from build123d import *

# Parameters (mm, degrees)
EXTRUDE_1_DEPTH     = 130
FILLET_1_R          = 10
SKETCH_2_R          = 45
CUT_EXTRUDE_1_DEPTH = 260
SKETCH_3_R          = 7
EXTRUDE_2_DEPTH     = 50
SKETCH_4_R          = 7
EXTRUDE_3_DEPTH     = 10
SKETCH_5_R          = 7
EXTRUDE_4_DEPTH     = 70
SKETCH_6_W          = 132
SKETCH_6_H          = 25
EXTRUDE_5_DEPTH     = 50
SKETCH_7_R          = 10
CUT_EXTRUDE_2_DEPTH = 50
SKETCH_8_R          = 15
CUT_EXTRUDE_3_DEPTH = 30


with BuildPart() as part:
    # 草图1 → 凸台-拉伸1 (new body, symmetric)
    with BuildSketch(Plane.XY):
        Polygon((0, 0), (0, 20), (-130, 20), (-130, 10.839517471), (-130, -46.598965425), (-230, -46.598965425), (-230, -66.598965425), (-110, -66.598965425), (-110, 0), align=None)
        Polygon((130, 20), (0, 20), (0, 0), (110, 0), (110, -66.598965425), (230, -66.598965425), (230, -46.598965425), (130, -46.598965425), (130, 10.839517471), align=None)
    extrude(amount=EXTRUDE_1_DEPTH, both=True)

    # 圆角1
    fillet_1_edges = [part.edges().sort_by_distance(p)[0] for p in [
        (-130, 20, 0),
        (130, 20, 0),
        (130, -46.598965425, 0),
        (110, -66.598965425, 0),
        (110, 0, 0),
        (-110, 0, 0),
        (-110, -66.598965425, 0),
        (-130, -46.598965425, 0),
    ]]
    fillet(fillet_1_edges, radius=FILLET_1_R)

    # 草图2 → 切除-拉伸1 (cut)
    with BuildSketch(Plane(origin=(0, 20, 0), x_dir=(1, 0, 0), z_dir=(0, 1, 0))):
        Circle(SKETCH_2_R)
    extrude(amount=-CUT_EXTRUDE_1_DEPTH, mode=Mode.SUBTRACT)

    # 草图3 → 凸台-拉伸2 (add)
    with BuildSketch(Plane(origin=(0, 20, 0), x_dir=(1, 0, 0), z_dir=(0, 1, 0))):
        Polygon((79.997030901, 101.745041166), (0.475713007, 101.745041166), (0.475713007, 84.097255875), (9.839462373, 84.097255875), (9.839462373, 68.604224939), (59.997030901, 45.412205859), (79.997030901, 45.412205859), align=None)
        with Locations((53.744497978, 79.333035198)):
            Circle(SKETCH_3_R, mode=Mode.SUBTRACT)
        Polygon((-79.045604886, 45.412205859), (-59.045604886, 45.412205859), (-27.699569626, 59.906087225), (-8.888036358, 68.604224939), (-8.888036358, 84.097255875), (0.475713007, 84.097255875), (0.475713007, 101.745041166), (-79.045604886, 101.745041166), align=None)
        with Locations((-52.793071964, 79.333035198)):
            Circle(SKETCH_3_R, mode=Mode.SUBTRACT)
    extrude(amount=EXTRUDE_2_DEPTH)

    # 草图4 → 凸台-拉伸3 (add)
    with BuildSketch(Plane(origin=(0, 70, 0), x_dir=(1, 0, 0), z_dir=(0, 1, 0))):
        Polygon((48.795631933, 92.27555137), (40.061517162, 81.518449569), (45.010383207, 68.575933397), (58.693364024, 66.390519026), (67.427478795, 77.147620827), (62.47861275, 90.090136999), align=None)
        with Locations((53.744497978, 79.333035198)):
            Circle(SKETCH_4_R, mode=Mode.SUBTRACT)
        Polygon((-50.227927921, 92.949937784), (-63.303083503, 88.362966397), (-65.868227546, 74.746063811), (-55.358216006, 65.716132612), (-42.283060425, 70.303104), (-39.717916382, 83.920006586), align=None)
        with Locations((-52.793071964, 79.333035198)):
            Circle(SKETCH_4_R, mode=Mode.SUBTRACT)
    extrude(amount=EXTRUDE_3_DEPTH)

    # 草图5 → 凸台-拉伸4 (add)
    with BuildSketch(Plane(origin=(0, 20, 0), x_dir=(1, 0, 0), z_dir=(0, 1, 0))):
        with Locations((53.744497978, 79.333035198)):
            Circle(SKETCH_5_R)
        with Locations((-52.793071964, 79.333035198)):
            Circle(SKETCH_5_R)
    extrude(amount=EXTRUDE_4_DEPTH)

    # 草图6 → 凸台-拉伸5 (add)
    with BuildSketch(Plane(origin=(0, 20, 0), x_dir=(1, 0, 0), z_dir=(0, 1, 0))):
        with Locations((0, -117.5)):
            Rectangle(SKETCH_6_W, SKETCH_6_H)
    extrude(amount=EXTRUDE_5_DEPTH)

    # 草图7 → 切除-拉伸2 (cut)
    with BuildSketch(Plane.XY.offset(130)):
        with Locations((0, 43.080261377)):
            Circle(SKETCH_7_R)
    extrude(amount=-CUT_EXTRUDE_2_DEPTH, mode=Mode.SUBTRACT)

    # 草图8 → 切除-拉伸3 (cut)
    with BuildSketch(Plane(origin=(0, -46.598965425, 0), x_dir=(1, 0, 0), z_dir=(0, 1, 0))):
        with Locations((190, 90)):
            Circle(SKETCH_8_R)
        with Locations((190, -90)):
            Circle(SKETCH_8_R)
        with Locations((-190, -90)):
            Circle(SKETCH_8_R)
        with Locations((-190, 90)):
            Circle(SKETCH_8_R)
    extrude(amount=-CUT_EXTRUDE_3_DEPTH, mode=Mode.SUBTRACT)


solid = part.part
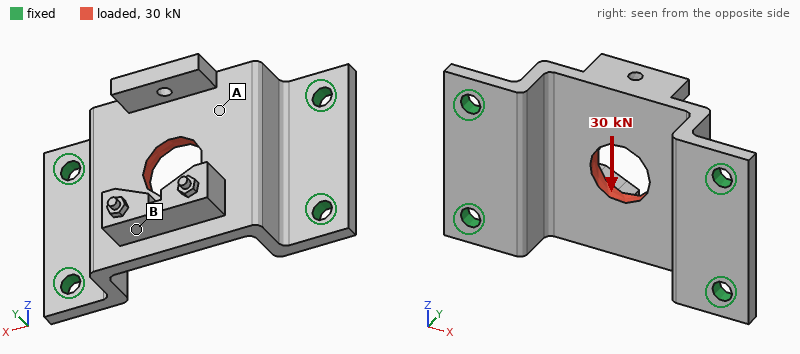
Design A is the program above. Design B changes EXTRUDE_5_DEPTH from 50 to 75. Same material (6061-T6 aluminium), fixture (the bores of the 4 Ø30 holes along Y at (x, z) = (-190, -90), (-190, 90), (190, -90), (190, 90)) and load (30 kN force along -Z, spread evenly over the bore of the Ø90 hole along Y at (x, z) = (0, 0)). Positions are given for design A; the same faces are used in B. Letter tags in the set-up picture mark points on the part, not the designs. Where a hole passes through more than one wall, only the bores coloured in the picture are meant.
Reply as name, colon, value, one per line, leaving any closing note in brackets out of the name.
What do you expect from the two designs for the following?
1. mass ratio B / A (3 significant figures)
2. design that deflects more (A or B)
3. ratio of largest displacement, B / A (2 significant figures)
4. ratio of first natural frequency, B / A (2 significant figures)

mass ratio B / A: 1.02
design that deflects more: B
ratio of largest displacement, B / A: 1.1
ratio of first natural frequency, B / A: 0.93
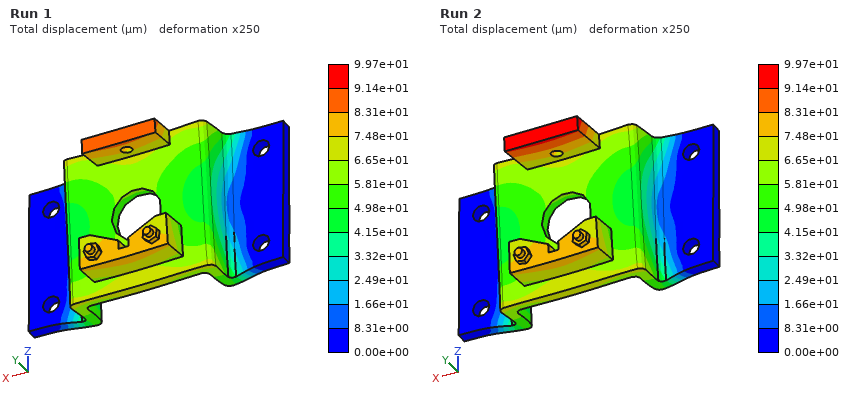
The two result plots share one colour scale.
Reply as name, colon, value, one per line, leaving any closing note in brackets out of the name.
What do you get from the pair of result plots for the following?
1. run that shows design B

run that shows design B: Run 2
